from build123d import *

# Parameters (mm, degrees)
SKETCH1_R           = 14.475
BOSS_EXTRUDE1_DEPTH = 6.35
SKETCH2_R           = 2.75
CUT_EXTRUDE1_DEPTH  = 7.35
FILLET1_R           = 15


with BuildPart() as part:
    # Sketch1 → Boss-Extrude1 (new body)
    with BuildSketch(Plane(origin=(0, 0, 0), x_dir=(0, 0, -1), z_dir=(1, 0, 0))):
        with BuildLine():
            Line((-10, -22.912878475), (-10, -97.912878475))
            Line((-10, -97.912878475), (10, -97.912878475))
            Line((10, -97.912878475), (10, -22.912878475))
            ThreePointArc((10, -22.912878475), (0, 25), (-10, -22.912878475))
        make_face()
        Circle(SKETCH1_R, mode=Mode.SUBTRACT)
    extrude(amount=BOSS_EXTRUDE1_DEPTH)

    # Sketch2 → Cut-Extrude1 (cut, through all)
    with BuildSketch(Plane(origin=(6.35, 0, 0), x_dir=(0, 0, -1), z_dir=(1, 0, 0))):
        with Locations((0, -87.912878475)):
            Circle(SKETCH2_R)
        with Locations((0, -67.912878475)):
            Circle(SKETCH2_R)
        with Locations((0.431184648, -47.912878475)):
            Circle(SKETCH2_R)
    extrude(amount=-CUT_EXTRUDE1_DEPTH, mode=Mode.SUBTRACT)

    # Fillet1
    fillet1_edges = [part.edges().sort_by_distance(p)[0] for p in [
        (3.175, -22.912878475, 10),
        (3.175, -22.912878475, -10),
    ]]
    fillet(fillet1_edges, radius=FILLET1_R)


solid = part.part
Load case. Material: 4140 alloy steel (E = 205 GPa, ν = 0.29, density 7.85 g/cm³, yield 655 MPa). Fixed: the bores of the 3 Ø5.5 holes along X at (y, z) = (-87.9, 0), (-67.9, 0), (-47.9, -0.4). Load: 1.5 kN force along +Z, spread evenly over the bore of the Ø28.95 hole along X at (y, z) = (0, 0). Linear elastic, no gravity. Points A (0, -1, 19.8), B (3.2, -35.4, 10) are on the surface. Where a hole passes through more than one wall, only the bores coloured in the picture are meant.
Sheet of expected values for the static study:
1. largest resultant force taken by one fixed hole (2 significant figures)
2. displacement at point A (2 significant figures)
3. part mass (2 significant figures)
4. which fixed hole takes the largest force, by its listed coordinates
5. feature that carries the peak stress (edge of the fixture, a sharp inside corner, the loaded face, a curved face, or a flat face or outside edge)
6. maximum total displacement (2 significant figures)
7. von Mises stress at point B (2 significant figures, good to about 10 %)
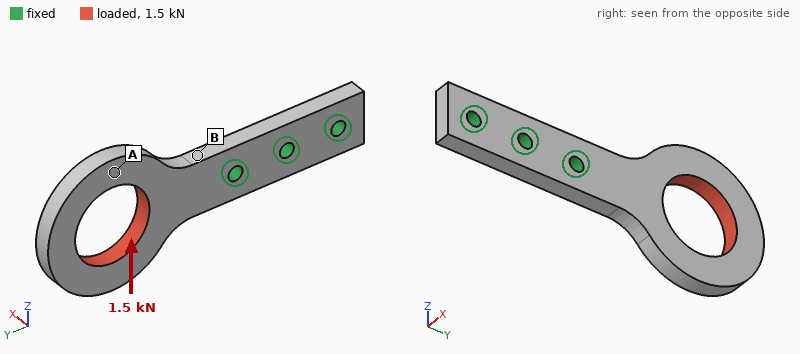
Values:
3.4 kN
0.11 mm
140 g
(-47.9, -0.4)
edge of the fixture
0.17 mm
130 MPa
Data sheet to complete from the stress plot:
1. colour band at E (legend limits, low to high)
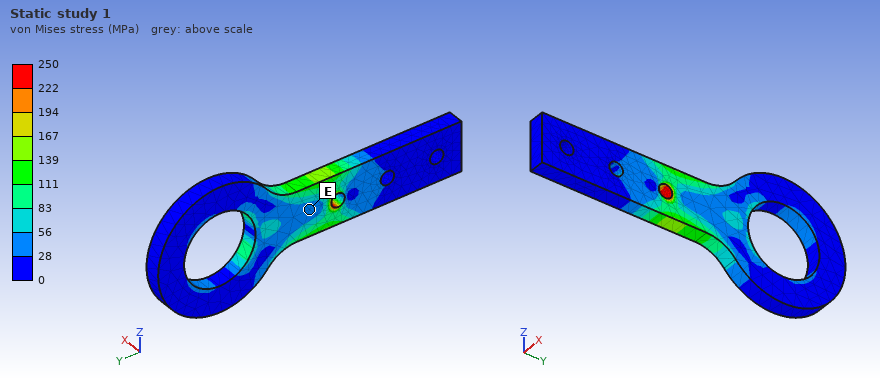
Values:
28 to 56 MPa
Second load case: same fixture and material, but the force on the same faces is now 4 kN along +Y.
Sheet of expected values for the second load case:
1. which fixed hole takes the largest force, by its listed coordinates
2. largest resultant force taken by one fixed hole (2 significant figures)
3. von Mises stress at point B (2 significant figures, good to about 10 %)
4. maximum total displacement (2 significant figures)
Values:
(-47.9, -0.4)
3.5 kN
29 MPa
19 µm
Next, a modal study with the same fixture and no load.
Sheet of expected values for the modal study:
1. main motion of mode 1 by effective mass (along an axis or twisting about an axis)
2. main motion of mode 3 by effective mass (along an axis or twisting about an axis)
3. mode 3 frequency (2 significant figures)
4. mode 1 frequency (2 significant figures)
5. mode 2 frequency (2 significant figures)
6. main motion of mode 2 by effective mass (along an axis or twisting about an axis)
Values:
along X
twisting about Y
2300 Hz
870 Hz
2100 Hz
along Z
